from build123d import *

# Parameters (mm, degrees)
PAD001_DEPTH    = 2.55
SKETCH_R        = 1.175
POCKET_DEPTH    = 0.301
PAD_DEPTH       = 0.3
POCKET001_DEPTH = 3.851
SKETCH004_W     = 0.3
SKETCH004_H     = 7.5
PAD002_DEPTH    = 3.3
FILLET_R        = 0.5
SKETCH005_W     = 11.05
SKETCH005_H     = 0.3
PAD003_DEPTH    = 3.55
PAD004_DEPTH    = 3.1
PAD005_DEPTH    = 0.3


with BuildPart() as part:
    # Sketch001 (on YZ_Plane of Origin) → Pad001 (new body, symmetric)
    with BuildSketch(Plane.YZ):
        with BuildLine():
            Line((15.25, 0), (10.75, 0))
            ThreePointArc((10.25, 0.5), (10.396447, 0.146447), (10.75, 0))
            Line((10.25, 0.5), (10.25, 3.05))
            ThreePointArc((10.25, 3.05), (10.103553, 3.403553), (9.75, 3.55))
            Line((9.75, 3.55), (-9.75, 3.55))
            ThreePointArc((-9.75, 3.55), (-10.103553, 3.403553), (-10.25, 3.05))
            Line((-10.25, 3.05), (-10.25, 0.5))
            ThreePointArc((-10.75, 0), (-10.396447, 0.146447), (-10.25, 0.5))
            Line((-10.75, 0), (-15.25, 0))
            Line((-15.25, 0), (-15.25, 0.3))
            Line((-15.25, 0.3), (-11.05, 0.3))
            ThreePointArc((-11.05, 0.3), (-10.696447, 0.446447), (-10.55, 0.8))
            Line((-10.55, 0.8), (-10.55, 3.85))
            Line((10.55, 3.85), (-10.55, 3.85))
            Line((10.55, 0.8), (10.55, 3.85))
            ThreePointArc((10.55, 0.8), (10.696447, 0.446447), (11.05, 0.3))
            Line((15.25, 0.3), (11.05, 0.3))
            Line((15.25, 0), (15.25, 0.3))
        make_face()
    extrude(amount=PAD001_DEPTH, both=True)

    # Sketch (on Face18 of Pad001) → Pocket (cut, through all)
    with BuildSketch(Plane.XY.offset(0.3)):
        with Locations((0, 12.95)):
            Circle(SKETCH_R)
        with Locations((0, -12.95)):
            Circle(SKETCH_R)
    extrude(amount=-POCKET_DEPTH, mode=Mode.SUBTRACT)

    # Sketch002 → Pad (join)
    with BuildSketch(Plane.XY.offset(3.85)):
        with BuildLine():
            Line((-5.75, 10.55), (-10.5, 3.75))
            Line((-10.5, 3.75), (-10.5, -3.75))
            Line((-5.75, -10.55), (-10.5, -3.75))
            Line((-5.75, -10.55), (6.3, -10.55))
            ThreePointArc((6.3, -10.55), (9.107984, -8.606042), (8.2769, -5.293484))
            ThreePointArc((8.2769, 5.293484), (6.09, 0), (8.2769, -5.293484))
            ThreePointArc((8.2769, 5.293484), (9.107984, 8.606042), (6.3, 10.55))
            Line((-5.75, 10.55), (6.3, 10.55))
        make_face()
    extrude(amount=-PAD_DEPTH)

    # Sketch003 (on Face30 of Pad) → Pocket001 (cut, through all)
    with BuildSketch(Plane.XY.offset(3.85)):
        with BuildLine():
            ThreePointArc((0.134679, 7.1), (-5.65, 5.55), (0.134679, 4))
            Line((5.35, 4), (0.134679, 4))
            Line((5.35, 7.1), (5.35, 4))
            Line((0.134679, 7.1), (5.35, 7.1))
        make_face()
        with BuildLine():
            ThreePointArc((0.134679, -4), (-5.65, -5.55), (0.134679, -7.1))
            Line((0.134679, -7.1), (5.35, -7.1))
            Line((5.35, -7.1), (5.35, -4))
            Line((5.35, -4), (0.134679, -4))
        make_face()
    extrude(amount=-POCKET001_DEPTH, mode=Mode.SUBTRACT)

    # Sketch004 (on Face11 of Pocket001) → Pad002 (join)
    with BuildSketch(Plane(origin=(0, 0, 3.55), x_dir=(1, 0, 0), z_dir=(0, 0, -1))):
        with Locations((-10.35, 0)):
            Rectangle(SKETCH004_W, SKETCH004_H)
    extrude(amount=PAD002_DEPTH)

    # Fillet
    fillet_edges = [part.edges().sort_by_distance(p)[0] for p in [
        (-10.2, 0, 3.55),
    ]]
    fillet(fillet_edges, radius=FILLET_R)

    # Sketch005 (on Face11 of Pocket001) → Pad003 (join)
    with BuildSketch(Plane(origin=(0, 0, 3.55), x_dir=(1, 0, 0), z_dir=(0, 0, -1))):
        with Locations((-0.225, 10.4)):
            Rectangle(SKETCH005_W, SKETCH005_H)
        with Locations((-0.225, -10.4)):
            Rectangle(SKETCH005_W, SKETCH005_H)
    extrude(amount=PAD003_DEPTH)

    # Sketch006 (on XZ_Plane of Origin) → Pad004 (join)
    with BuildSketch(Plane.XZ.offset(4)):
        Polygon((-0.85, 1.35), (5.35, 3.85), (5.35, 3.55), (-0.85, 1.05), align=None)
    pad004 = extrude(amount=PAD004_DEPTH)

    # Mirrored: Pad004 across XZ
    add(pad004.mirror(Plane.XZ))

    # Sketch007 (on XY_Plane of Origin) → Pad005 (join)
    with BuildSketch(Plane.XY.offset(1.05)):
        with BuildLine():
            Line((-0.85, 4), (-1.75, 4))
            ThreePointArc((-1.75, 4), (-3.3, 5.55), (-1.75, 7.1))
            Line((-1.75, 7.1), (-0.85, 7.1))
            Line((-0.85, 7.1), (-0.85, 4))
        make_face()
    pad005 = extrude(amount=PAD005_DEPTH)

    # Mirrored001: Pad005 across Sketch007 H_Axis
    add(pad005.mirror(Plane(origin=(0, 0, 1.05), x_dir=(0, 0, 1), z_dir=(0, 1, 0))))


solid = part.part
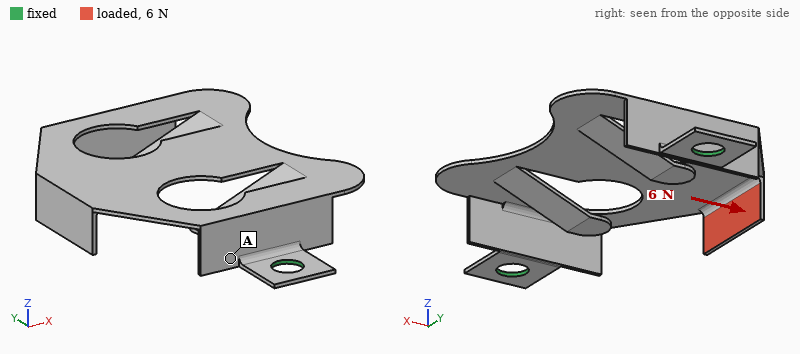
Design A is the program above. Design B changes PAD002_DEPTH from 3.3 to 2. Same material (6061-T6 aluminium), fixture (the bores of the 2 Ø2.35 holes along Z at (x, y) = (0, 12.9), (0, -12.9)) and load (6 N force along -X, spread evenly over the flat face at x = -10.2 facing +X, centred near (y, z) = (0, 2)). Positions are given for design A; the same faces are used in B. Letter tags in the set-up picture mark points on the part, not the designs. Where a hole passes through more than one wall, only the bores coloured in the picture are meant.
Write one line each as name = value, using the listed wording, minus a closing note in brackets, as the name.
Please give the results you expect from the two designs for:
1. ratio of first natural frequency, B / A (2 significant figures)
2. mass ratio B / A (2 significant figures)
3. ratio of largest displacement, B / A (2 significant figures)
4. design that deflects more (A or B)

ratio of first natural frequency, B / A = 1.1
mass ratio B / A = 0.98
ratio of largest displacement, B / A = 0.53
design that deflects more = A
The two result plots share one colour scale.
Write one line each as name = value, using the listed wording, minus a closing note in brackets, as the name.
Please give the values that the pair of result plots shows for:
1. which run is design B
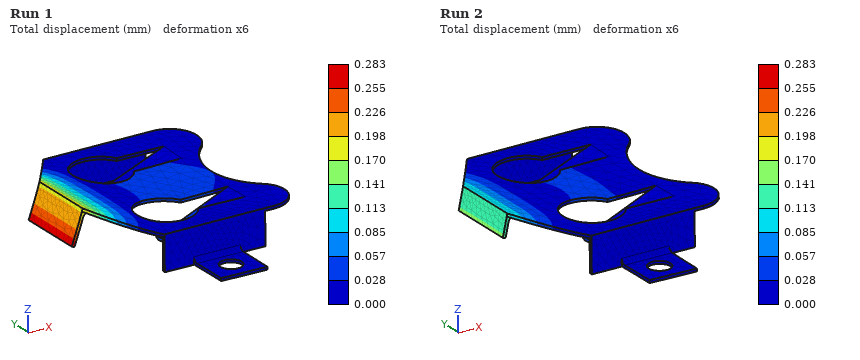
which run is design B = Run 2
